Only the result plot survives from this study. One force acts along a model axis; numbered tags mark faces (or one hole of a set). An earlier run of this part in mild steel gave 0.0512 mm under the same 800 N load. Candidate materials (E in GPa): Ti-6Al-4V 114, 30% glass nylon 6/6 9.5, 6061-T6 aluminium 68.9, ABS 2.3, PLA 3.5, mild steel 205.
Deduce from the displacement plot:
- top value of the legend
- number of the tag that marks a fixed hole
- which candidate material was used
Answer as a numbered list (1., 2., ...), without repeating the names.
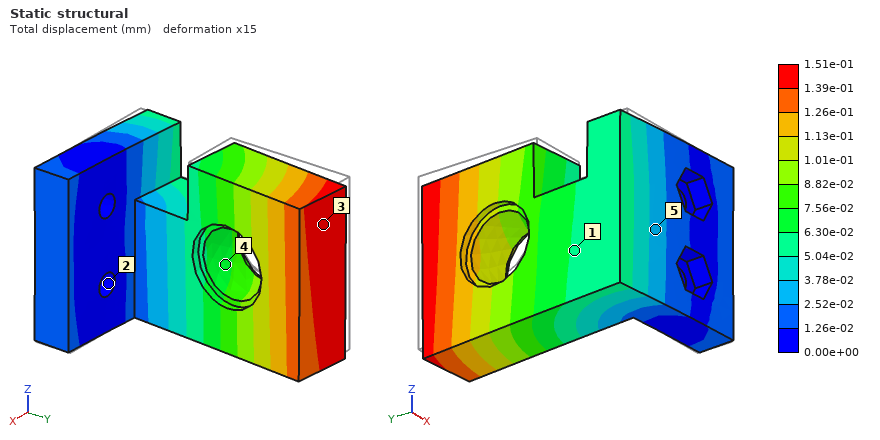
1. 1.51e-01 mm
2. 2
3. 6061-T6 aluminium
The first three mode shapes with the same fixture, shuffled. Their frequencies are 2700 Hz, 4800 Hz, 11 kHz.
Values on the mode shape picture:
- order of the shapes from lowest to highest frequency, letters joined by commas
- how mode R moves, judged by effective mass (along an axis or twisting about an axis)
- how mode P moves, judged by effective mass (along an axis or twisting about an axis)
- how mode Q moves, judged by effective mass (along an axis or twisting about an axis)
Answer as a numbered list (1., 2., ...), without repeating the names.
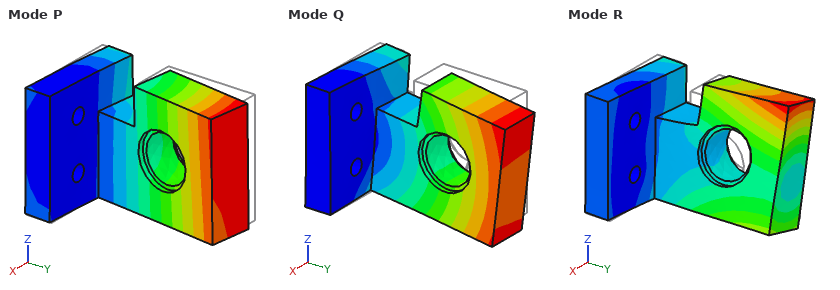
1. P, Q, R
2. along Y
3. along X
4. along Z
